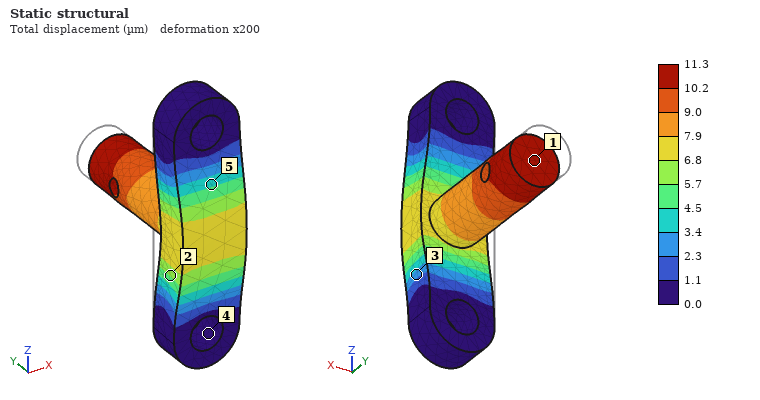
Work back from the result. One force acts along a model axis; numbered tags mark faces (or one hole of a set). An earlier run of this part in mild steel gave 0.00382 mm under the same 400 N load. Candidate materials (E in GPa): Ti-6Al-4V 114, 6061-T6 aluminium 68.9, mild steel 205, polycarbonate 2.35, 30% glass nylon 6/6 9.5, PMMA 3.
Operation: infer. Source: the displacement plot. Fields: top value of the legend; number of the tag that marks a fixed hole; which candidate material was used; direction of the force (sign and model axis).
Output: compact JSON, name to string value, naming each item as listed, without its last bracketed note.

{"top value of the legend": "11.3 µm", "number of the tag that marks a fixed hole": "4", "which candidate material was used": "6061-T6 aluminium", "direction of the force": "-Y"}
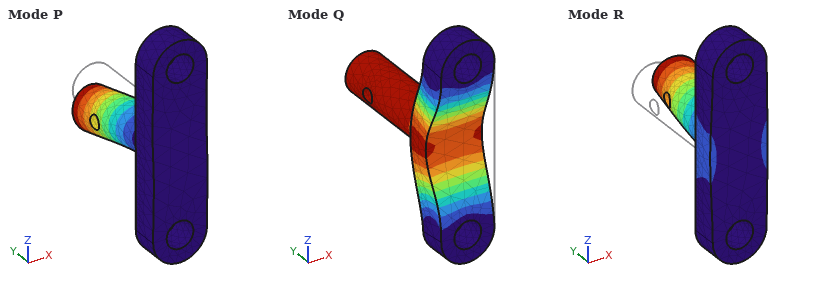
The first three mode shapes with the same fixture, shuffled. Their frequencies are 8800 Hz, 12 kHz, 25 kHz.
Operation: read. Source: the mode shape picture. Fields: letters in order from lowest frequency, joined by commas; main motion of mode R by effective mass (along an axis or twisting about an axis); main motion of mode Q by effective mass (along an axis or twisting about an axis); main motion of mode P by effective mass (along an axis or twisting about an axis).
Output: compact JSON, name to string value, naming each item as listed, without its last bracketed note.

{"letters in order from lowest frequency, joined by commas": "R, P, Q", "main motion of mode R by effective mass": "along X", "main motion of mode Q by effective mass": "along Y", "main motion of mode P by effective mass": "along Z"}
